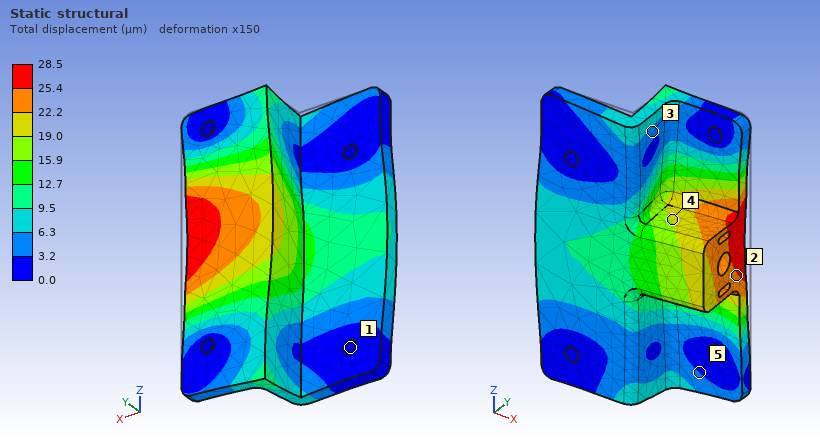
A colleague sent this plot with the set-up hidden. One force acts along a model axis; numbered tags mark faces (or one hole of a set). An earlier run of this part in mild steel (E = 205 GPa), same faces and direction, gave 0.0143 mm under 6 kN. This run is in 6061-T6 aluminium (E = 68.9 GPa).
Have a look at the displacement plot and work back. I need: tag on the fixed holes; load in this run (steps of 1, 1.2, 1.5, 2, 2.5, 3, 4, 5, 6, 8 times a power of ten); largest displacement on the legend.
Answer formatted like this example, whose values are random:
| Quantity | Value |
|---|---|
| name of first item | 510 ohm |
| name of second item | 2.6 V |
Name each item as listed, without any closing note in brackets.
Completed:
| Quantity | Value |
|---|---|
| tag on the fixed holes | 1 |
| load in this run | 4 kN |
| largest displacement on the legend | 28.5 µm |
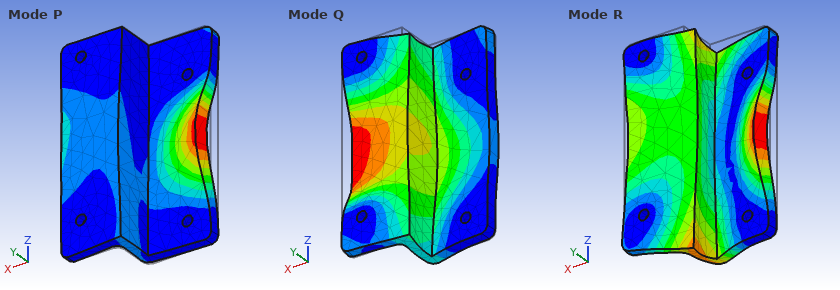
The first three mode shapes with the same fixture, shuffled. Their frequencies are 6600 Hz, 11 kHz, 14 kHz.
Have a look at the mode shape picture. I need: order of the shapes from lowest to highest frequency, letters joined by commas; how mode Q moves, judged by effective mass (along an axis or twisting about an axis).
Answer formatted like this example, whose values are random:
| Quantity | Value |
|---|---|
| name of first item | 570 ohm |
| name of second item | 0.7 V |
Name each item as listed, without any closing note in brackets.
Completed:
| Quantity | Value |
|---|---|
| order of the shapes from lowest to highest frequency, letters joined by commas | Q, P, R |
| how mode Q moves, judged by effective mass | along Y |
